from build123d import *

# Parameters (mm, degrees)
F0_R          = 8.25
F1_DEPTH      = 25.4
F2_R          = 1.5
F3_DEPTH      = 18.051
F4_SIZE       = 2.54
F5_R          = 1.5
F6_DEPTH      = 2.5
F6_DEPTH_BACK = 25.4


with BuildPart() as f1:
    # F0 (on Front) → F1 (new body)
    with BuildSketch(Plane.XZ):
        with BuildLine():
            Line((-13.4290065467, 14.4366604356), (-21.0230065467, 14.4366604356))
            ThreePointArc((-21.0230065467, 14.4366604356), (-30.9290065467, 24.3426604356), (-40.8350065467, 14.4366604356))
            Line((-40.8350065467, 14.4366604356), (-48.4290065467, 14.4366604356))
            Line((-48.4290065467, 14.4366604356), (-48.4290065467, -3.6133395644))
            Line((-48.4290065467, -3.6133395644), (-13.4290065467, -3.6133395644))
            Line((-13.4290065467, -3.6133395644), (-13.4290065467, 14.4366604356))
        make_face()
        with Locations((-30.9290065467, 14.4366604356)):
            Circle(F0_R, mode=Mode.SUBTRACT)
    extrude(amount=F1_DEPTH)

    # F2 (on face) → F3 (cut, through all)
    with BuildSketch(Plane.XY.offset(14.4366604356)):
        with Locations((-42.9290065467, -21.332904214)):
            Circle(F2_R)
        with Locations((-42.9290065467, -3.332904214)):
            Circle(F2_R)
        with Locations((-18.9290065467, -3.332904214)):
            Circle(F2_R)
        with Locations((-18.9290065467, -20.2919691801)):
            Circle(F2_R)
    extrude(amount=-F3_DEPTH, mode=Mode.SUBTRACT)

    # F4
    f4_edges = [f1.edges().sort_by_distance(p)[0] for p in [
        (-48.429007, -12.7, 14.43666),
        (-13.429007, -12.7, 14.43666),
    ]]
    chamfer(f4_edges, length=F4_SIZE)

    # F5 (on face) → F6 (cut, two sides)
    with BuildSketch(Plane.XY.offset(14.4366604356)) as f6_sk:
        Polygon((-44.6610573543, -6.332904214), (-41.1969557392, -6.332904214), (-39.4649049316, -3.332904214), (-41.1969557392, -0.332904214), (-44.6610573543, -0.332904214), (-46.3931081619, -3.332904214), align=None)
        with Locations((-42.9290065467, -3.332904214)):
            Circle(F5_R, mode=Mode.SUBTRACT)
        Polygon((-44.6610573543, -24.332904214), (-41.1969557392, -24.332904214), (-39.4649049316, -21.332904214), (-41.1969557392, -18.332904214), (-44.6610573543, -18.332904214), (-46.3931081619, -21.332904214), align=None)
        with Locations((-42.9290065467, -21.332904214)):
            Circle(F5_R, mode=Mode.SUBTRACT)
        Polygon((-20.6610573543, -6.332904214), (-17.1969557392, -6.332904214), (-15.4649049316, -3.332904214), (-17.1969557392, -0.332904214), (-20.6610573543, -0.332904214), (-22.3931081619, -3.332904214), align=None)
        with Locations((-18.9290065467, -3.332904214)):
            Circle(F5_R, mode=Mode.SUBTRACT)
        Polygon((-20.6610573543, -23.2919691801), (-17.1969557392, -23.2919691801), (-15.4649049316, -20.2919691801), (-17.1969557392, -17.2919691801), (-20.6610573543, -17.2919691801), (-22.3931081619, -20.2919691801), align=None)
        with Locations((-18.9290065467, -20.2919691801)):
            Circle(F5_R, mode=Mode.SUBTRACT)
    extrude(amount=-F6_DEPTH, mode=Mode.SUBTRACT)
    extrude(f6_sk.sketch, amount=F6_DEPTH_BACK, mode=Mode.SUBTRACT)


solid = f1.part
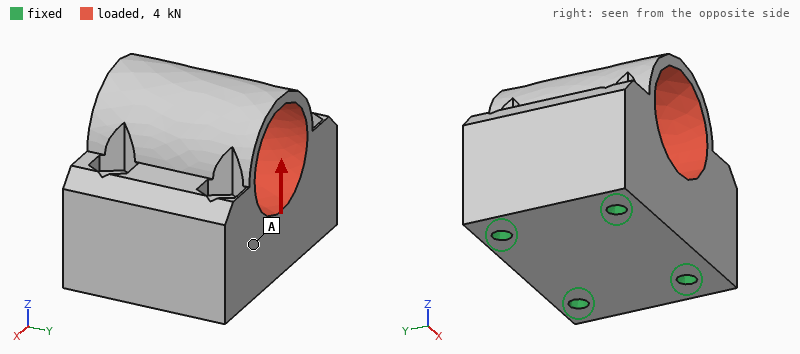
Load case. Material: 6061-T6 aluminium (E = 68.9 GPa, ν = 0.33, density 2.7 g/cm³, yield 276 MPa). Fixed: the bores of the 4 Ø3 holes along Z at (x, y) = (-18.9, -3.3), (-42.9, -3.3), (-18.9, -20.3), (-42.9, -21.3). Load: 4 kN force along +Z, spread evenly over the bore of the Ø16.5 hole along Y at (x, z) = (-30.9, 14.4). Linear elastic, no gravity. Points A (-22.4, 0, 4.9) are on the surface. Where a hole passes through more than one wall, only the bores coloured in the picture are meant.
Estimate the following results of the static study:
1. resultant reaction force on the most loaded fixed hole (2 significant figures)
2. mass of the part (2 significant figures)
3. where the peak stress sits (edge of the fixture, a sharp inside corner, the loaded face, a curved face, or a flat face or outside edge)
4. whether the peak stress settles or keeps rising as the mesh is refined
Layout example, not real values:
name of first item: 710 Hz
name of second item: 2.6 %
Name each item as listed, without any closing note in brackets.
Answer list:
resultant reaction force on the most loaded fixed hole: 1.1 kN
mass of the part: 37 g
where the peak stress sits: a sharp inside corner
whether the peak stress settles or keeps rising as the mesh is refined: keeps rising
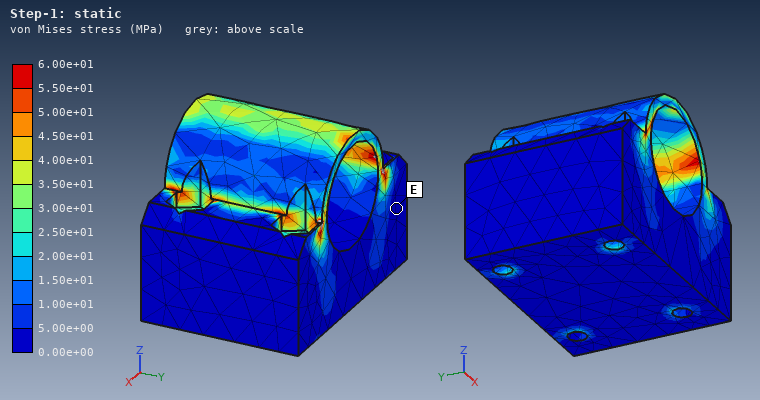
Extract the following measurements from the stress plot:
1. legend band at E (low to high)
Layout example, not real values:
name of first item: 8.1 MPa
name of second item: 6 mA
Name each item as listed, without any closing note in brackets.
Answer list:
legend band at E: 0.00e+00 to 5.00e+00 MPa
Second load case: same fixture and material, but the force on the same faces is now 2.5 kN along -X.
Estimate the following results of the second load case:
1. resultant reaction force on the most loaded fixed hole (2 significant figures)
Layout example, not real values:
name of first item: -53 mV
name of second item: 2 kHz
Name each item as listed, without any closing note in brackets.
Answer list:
resultant reaction force on the most loaded fixed hole: 760 N
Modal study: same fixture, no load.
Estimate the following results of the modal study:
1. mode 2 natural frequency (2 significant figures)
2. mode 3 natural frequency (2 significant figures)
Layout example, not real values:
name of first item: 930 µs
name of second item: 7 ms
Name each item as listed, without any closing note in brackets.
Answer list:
mode 2 natural frequency: 28 kHz
mode 3 natural frequency: 28 kHz
